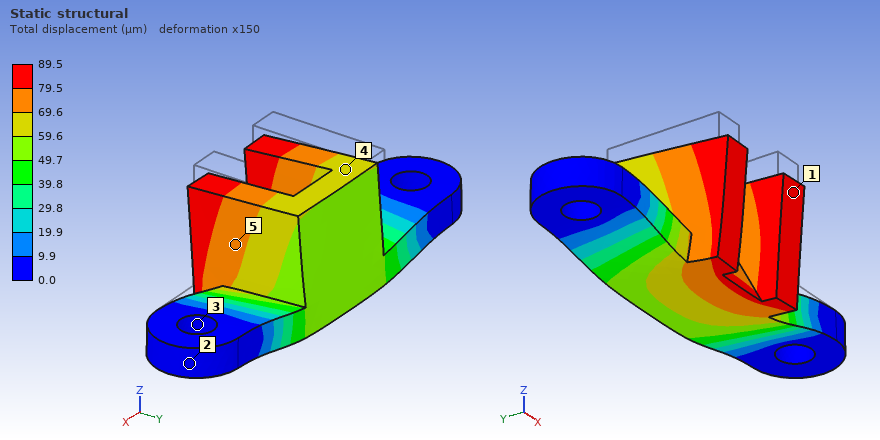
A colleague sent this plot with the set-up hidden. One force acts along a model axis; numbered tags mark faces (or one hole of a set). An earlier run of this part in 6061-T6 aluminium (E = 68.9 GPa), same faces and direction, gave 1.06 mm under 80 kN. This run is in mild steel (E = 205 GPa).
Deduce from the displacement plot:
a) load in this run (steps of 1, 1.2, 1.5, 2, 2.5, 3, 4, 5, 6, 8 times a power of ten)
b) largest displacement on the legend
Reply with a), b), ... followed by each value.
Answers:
a) 20 kN
b) 89.5 µm
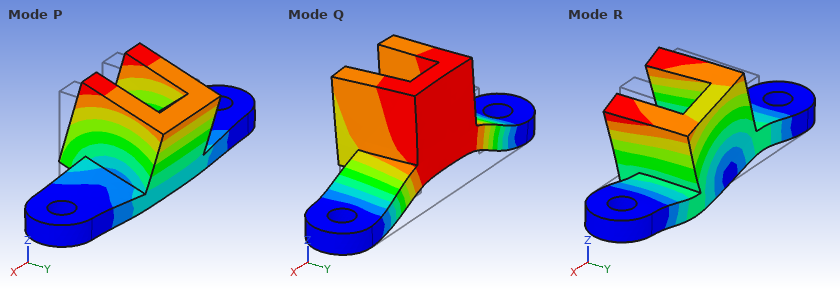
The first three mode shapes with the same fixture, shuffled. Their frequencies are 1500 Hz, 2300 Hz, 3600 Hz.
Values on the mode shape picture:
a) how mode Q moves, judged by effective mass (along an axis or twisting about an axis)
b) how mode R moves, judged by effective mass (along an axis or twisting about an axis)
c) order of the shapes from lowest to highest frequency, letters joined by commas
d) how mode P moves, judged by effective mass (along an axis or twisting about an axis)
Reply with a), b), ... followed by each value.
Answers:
a) along Z
b) along X
c) P, Q, R
d) along Y
